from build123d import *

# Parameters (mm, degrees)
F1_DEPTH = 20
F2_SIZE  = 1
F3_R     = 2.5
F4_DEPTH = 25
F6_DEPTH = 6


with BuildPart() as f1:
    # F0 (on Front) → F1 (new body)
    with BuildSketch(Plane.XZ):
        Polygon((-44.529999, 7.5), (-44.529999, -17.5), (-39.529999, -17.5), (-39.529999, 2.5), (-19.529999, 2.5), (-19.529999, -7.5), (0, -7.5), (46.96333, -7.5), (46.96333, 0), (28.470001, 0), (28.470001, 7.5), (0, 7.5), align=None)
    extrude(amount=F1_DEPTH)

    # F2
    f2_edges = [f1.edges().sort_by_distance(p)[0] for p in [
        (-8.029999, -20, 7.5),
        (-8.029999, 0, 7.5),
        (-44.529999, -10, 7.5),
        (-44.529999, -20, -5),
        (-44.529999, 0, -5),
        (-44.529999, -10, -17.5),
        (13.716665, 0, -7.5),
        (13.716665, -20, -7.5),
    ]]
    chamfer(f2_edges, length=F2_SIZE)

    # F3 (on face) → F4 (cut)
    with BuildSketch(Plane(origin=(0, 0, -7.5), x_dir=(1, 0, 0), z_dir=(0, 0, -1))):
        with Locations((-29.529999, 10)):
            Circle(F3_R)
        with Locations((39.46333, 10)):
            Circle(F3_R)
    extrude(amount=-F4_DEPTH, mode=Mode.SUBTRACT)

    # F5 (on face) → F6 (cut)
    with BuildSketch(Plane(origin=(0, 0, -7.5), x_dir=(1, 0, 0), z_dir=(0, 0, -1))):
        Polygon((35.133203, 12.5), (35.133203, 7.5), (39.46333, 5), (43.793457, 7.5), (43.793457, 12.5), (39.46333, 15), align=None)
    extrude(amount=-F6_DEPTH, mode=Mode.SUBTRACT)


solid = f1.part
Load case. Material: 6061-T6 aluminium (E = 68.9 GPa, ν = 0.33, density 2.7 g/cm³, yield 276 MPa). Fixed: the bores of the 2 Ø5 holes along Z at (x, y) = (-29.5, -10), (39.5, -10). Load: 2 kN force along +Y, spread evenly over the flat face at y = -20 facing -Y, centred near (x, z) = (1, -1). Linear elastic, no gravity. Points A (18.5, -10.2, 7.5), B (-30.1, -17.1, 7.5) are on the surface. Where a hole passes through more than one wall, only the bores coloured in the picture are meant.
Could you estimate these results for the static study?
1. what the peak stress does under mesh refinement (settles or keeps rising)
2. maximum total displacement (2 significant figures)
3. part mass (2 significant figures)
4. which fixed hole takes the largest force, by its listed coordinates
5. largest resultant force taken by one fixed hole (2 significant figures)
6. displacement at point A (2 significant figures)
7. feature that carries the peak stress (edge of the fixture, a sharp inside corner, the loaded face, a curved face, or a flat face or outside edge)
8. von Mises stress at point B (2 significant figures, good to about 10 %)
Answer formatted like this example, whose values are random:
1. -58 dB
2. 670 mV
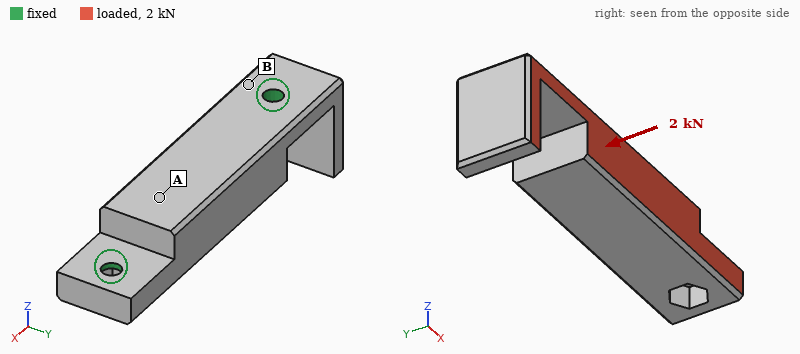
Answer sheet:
1. keeps rising
2. 29 µm
3. 57 g
4. (-29.5, -10)
5. 1.1 kN
6. 5.4 µm
7. edge of the fixture
8. 23 MPa
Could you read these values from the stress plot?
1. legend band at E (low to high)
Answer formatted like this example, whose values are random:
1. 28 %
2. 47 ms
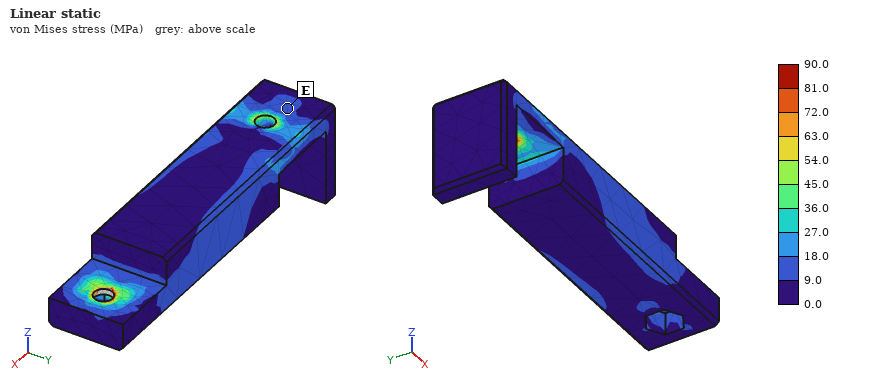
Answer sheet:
1. 9.0 to 18.0 MPa
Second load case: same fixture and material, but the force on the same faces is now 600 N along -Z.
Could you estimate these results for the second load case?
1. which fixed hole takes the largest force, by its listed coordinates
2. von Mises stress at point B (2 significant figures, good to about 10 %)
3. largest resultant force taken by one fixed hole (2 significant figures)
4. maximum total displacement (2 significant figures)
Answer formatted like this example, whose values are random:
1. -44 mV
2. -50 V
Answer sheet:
1. (-29.5, -10)
2. 22 MPa
3. 390 N
4. 28 µm
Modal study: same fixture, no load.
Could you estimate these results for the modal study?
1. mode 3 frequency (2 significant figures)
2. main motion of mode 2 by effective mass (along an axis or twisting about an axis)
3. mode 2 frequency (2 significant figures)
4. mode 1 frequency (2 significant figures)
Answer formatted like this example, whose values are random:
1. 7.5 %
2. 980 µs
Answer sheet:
1. 6200 Hz
2. along Y
3. 5400 Hz
4. 4500 Hz
